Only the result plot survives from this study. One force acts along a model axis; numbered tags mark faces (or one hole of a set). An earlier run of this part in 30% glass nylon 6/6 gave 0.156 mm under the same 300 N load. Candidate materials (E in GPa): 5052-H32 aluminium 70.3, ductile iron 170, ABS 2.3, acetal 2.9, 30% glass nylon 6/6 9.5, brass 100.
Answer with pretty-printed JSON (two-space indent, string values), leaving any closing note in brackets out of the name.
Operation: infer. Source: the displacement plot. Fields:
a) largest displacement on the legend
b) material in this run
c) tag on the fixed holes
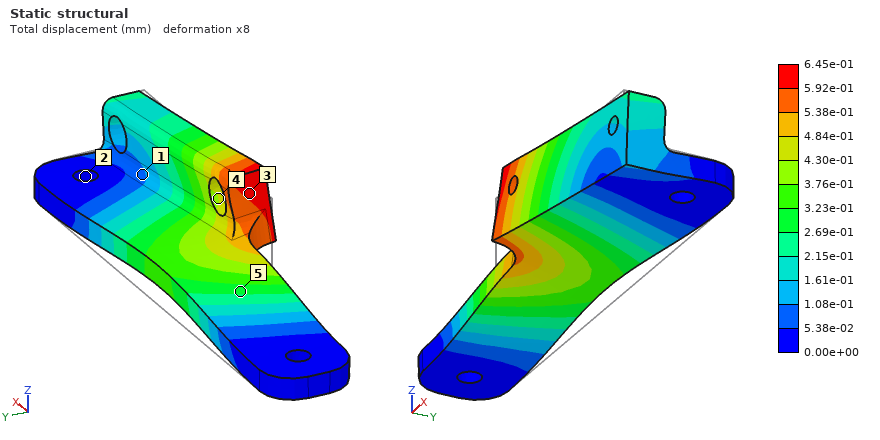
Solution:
{
  "largest displacement on the legend": "6.45e-01 mm",
  "material in this run": "ABS",
  "tag on the fixed holes": "2"
}
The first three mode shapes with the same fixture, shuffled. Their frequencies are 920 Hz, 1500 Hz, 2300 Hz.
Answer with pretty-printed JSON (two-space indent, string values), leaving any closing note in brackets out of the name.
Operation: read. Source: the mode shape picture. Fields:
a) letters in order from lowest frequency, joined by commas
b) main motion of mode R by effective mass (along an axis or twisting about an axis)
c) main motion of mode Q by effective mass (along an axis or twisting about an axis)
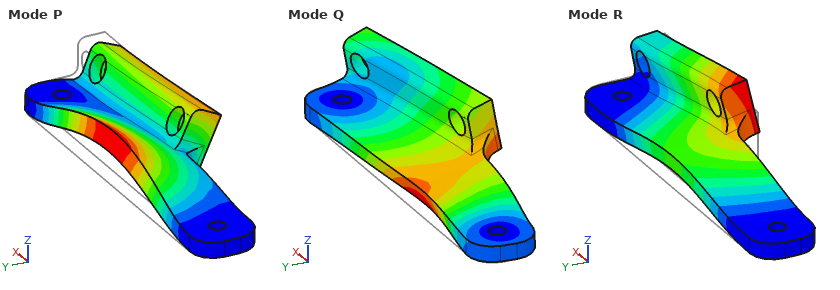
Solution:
{
  "letters in order from lowest frequency, joined by commas": "R, P, Q",
  "main motion of mode R by effective mass": "along Z",
  "main motion of mode Q by effective mass": "along Y"
}
